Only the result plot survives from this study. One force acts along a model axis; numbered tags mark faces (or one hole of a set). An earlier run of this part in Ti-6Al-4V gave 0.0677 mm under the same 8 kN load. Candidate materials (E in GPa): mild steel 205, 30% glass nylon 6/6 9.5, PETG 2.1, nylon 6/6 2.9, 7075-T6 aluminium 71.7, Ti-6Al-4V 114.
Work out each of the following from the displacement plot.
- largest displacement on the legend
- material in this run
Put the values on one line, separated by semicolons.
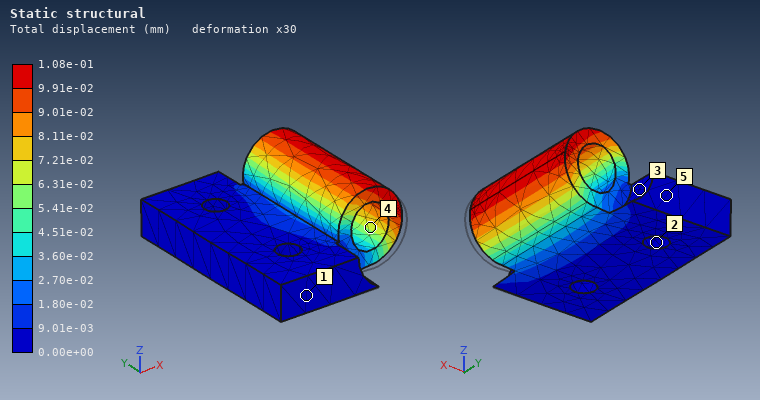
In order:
1.08e-01 mm; 7075-T6 aluminium
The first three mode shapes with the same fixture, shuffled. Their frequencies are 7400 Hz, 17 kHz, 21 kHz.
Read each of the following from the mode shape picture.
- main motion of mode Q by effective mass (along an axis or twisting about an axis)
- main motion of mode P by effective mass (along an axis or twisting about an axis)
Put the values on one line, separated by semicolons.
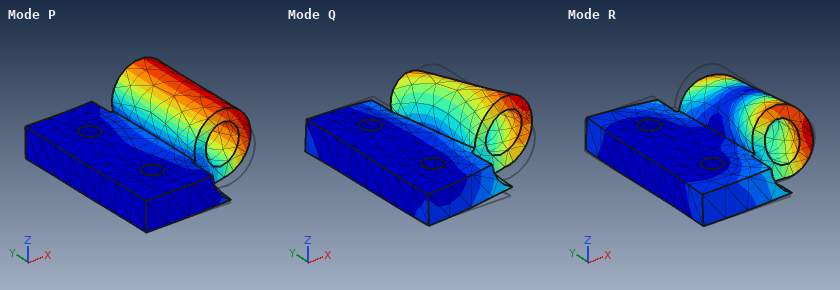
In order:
along Y; along Z
